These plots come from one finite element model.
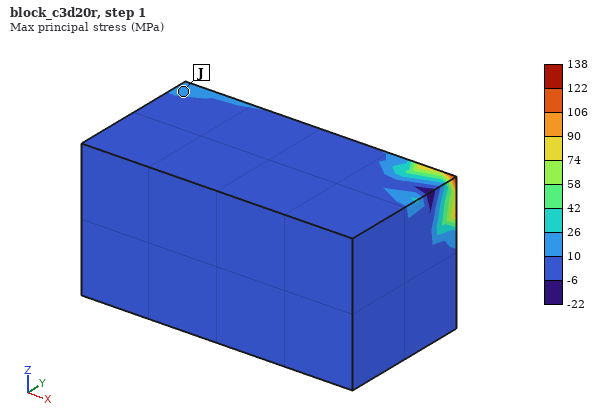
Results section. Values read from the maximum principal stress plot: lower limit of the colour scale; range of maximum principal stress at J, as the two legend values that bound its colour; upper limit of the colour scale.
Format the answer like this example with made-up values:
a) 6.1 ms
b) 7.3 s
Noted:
a) -22 MPa
b) 10 to 26 MPa
c) 138 MPa
